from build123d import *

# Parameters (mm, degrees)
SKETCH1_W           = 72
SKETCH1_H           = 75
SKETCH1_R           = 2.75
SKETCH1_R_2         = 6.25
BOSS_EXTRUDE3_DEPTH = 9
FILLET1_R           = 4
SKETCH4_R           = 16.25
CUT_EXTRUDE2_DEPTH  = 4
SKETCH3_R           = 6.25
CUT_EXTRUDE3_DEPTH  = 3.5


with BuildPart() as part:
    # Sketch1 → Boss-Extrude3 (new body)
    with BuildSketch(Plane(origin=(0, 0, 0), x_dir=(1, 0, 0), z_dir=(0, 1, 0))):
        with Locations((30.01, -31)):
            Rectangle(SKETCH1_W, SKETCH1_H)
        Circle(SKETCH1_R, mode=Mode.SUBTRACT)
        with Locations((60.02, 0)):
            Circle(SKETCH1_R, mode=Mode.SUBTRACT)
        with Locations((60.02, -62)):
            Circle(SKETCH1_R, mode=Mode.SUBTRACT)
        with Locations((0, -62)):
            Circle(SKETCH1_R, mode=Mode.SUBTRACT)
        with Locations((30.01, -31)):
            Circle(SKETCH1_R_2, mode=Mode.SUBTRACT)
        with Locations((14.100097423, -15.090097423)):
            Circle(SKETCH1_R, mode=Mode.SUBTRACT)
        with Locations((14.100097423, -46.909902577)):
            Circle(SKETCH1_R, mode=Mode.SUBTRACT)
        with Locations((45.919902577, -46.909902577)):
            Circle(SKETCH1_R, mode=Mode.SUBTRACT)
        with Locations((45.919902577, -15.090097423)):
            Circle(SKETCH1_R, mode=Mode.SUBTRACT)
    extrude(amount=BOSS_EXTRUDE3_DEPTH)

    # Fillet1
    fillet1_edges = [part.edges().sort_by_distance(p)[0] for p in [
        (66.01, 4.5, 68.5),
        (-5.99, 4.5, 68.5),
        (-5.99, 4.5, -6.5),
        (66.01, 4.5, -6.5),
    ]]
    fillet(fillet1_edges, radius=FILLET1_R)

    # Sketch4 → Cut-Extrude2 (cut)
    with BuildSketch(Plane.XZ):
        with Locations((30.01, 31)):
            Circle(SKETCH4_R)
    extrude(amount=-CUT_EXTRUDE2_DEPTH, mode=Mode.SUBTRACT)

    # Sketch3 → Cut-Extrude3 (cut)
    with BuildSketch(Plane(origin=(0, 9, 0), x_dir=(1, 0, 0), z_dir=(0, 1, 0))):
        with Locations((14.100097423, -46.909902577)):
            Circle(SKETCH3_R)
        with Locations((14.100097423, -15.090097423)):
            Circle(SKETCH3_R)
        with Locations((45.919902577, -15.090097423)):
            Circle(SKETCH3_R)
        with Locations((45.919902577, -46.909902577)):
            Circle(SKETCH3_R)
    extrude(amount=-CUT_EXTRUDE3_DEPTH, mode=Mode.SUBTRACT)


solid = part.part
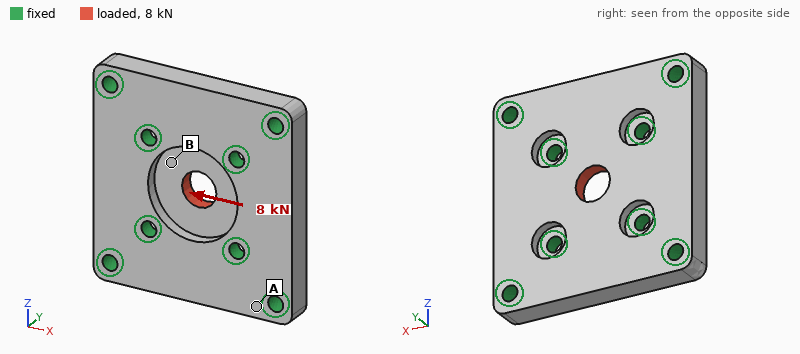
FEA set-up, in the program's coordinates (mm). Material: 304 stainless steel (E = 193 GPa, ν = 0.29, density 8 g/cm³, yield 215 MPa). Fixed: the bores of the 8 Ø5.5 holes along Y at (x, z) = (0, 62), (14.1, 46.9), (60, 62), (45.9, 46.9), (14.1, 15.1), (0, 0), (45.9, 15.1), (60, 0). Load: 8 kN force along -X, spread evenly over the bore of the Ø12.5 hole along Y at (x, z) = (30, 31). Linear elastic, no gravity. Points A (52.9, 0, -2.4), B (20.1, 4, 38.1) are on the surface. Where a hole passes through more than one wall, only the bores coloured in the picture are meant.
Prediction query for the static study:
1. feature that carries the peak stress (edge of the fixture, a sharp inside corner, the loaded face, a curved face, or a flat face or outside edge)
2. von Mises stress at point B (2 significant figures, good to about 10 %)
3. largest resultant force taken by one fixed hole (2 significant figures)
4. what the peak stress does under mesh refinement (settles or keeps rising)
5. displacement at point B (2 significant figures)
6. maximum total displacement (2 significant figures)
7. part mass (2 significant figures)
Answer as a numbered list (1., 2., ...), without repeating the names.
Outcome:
1. edge of the fixture
2. 37 MPa
3. 1.7 kN
4. keeps rising
5. 2.4 µm
6. 4.2 µm
7. 330 g
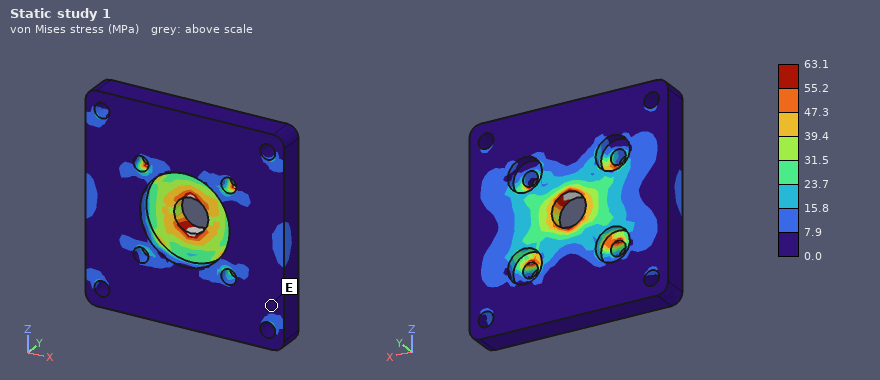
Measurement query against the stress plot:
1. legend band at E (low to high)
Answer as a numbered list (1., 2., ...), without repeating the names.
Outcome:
1. 0.0 to 7.9 MPa
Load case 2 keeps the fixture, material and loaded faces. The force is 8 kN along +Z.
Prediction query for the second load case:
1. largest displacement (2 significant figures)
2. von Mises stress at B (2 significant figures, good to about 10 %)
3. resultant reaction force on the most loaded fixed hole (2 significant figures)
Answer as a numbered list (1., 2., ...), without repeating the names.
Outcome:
1. 4.1 µm
2. 37 MPa
3. 1.7 kN
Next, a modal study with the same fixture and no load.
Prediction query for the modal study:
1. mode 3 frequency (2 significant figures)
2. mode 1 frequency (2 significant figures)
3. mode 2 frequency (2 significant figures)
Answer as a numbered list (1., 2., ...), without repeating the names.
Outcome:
1. 16 kHz
2. 15 kHz
3. 16 kHz
